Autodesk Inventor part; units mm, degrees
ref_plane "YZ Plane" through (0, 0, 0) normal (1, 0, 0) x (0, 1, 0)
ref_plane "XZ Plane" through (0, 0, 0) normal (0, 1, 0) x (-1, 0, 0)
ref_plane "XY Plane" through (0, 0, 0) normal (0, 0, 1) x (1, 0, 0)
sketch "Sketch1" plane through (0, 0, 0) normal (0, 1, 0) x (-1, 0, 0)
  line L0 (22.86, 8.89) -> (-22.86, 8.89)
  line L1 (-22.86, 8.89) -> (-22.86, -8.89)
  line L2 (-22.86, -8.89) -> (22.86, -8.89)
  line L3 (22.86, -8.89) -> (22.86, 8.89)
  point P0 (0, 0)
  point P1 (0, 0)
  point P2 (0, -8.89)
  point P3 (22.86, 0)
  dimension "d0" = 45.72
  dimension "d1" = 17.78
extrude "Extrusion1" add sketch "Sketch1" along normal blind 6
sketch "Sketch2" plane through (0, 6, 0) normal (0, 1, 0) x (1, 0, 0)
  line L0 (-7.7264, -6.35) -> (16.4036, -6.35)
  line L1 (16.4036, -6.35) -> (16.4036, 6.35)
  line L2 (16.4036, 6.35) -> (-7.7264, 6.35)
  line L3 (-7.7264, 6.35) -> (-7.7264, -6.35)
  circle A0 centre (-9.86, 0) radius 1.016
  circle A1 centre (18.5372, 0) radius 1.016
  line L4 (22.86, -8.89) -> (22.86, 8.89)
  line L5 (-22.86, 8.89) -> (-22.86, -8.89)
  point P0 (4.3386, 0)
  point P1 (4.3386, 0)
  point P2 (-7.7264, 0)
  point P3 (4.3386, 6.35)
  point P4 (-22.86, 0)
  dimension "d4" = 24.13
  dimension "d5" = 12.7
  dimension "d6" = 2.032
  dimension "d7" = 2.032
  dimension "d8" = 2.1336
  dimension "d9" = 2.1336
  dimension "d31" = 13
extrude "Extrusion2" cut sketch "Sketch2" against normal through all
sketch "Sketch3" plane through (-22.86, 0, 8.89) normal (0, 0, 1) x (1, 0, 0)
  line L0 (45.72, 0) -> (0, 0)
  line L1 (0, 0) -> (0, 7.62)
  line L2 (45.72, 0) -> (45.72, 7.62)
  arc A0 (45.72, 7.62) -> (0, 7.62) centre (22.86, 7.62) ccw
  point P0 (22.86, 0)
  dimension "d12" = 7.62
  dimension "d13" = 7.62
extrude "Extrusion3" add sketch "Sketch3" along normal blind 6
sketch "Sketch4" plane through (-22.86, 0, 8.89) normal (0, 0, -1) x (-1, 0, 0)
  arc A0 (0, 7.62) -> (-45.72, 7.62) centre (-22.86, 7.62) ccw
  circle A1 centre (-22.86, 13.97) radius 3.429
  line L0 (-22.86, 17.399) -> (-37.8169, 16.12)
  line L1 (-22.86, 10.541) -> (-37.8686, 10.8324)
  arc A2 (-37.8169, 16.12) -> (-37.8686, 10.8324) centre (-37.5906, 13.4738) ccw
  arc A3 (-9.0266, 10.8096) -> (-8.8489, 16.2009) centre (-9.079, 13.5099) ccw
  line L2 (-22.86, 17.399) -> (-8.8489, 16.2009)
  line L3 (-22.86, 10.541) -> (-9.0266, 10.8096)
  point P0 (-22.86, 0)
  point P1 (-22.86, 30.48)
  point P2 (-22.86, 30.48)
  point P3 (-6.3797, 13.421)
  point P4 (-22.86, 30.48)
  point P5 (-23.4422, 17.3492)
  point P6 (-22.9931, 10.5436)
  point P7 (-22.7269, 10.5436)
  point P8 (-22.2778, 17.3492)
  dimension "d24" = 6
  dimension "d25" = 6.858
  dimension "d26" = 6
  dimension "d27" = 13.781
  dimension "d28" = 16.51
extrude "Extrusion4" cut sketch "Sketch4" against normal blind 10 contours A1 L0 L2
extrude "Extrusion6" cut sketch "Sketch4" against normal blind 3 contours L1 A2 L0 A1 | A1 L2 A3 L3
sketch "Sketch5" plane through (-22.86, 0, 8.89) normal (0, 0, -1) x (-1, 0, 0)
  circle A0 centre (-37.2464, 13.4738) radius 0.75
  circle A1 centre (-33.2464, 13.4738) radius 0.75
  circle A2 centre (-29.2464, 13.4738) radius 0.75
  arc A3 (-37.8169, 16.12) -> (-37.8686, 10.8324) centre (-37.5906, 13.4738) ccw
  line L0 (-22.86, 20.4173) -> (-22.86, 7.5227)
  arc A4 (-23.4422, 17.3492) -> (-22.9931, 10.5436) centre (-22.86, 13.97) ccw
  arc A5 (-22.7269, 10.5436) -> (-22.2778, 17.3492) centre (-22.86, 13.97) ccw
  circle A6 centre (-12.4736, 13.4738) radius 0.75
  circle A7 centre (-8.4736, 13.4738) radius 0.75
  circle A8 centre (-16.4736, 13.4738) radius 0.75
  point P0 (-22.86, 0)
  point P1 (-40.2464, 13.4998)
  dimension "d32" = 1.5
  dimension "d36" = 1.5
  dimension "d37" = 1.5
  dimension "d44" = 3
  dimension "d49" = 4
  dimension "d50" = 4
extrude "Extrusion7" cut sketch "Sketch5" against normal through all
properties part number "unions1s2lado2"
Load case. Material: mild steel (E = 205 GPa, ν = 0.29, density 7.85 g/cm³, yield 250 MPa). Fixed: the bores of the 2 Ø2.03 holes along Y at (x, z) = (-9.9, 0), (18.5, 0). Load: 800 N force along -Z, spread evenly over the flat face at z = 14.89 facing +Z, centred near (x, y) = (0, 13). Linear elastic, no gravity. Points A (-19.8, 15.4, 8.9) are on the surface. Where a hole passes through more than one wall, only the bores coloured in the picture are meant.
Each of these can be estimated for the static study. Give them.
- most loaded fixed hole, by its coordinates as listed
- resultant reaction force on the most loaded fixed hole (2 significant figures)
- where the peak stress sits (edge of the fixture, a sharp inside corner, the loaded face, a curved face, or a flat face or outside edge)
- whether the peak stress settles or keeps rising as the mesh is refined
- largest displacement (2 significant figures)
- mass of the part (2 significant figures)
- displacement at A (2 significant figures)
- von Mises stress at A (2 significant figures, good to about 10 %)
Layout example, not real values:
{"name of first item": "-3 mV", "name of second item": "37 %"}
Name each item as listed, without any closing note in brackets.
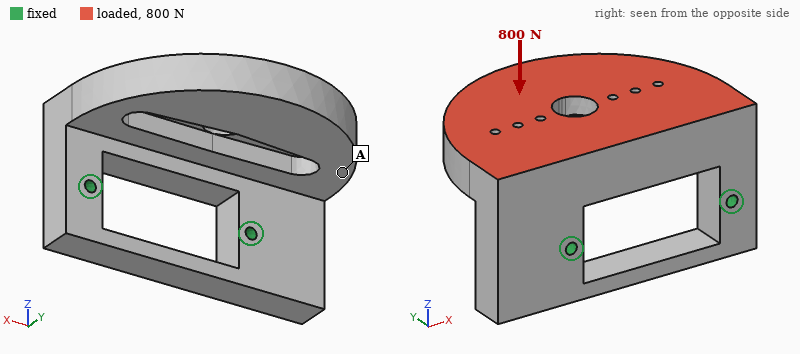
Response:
{"most loaded fixed hole, by its coordinates as listed": "(-9.9, 0)", "resultant reaction force on the most loaded fixed hole": "520 N", "where the peak stress sits": "edge of the fixture", "whether the peak stress settles or keeps rising as the mesh is refined": "keeps rising", "largest displacement": "56 µm", "mass of the part": "73 g", "displacement at A": "20 µm", "von Mises stress at A": "26 MPa"}
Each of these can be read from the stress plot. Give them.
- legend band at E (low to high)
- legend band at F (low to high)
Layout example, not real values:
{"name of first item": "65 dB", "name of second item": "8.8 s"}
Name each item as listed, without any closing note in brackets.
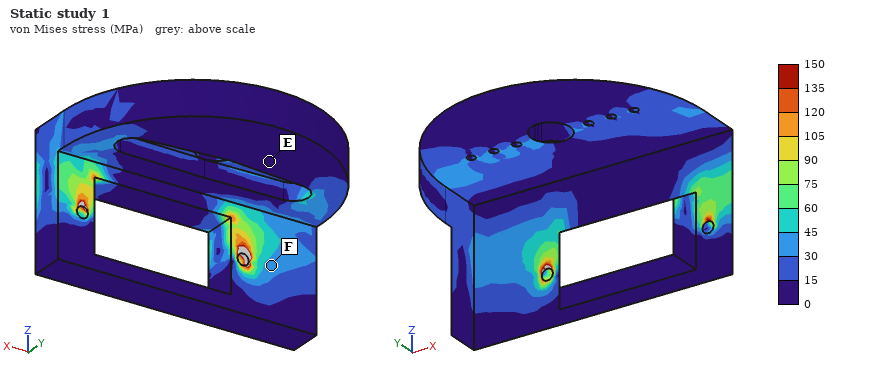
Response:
{"legend band at E": "0 to 15 MPa", "legend band at F": "30 to 45 MPa"}
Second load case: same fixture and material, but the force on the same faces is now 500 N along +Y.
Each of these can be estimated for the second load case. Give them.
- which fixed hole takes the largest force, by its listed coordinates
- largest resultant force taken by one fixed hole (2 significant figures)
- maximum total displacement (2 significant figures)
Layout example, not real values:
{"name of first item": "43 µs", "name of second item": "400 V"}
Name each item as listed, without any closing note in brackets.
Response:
{"which fixed hole takes the largest force, by its listed coordinates": "(-9.9, 0)", "largest resultant force taken by one fixed hole": "310 N", "maximum total displacement": "28 µm"}
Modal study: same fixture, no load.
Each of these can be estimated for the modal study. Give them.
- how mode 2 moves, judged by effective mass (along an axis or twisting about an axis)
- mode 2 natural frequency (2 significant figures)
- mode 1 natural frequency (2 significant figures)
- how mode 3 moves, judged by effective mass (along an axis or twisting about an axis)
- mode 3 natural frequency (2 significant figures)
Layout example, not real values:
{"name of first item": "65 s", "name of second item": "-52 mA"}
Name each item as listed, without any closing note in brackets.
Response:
{"how mode 2 moves, judged by effective mass": "along X", "mode 2 natural frequency": "6900 Hz", "mode 1 natural frequency": "3200 Hz", "how mode 3 moves, judged by effective mass": "along Y", "mode 3 natural frequency": "9100 Hz"}
